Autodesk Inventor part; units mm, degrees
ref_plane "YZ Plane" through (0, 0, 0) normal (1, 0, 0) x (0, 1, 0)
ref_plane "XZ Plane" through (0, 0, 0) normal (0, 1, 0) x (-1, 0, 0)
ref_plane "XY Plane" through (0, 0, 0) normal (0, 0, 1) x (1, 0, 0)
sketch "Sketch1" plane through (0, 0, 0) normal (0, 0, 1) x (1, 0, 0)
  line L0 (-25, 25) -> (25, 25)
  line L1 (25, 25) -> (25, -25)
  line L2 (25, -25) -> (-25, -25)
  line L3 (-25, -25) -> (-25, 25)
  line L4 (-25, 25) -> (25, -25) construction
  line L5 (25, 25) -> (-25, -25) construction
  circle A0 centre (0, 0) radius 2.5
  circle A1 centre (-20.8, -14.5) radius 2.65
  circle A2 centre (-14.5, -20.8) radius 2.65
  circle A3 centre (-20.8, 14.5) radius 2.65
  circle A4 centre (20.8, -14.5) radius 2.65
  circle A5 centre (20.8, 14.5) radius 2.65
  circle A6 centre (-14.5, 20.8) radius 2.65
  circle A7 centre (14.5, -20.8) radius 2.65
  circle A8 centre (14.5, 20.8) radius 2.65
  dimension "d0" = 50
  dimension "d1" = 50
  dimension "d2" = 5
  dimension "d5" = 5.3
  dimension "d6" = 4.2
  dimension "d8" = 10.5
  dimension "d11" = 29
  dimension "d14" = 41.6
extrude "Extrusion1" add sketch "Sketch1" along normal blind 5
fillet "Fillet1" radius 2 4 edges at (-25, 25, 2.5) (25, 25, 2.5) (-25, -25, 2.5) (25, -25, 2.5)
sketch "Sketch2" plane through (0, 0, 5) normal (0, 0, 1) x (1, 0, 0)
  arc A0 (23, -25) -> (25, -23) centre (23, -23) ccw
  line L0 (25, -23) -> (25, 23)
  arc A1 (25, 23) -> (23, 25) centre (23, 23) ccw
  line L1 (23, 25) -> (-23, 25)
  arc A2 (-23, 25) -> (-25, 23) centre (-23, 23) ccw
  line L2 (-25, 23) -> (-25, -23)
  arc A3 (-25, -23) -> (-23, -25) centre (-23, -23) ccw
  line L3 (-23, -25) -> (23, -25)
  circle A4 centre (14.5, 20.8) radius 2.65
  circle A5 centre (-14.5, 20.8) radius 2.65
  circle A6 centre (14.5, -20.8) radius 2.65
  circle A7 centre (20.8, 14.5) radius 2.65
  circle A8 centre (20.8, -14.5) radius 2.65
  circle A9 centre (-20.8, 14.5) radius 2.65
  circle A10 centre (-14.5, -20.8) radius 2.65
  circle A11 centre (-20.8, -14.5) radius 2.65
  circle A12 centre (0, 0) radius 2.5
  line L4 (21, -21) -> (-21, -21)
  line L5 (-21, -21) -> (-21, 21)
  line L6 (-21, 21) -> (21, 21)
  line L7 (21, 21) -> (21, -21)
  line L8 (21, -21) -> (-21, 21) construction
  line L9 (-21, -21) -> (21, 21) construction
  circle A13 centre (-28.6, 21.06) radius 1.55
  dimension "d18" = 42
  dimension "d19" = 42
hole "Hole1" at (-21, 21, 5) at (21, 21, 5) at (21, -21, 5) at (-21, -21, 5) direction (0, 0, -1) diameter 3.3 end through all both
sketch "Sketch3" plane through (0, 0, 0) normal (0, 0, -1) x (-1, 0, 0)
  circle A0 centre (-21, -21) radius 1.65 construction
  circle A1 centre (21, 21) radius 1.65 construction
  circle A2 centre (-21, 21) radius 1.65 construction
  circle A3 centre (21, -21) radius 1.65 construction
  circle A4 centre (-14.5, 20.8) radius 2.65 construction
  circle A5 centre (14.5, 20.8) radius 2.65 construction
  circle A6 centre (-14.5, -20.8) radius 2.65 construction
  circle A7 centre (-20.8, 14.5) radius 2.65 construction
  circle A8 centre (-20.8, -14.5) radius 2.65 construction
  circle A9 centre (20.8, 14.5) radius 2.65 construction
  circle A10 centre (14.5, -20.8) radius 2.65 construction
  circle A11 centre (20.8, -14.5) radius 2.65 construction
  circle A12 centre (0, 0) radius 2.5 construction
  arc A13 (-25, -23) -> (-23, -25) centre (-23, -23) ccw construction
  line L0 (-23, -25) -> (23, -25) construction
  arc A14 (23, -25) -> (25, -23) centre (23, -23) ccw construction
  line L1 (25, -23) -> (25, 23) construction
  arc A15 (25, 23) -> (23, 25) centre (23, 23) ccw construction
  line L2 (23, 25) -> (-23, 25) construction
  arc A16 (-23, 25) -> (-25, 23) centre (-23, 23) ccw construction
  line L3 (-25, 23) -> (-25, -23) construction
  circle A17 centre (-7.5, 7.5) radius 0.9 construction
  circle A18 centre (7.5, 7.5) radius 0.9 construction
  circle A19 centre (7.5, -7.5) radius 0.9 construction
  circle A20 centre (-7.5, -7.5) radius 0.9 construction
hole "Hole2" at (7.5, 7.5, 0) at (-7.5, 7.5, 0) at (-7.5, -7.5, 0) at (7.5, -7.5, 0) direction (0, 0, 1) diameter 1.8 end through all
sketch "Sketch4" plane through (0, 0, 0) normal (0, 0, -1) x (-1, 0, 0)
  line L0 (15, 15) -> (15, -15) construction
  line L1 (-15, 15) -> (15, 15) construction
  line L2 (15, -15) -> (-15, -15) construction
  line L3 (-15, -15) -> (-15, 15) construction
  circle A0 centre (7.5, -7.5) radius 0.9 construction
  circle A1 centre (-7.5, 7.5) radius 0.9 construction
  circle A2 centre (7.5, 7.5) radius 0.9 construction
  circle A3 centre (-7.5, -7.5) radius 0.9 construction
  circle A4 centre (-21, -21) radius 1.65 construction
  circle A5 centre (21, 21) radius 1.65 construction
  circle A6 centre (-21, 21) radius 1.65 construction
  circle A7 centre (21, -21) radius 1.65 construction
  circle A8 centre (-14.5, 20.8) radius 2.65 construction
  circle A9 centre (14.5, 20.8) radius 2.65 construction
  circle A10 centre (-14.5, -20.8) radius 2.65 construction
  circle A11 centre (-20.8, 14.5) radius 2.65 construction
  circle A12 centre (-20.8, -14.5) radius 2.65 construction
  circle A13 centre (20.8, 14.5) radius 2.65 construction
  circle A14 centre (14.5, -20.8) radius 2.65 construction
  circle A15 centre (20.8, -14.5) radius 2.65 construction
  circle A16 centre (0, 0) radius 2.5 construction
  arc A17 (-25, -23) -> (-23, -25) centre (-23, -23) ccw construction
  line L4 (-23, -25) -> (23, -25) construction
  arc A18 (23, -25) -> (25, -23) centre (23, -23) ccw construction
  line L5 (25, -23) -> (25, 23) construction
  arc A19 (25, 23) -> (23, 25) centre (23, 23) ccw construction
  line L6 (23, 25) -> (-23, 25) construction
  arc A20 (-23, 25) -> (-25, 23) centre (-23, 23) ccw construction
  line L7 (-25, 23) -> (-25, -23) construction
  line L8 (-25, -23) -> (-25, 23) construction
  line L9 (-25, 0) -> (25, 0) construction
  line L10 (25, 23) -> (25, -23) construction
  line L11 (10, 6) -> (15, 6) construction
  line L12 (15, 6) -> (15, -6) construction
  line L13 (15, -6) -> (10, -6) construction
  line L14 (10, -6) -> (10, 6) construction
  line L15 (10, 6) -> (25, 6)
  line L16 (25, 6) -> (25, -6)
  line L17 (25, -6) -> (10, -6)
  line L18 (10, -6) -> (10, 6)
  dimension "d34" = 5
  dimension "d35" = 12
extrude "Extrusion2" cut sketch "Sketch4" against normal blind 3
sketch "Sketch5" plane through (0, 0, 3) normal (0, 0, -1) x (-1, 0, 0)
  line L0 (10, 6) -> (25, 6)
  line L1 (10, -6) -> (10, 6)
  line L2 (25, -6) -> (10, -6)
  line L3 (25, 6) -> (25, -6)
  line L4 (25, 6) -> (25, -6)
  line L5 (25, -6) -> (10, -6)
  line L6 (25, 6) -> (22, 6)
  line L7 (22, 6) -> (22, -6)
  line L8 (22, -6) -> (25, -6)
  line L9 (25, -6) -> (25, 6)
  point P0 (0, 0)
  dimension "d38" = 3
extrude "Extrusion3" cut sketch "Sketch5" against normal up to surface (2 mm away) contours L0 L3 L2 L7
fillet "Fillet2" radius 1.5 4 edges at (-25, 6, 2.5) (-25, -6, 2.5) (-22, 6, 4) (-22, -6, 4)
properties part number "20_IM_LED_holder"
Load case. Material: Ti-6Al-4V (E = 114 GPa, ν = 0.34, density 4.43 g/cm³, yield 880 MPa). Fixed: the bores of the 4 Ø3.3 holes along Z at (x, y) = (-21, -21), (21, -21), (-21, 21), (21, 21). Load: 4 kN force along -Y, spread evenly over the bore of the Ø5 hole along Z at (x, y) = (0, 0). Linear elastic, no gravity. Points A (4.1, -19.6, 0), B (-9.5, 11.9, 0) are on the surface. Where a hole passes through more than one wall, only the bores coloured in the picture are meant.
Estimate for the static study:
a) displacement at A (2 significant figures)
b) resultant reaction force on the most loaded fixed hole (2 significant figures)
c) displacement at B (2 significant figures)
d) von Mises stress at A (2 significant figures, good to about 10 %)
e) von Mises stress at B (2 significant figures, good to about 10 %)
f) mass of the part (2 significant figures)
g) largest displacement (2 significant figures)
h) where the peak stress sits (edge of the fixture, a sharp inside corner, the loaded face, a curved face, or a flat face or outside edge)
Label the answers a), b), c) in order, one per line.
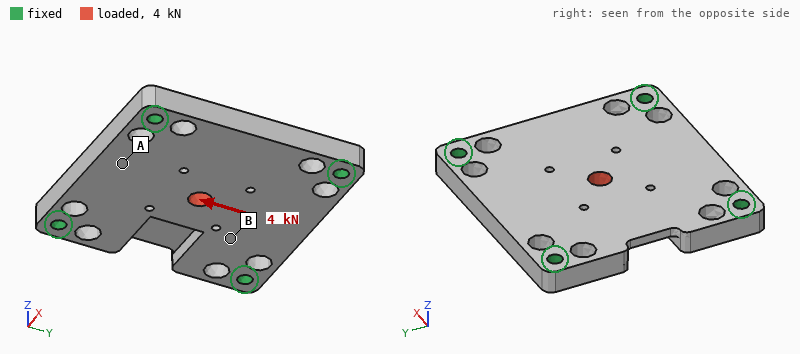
a) 6.2 µm
b) 1.2 kN
c) 5.6 µm
d) 8.9 MPa
e) 20 MPa
f) 47 g
g) 9.4 µm
h) the loaded face
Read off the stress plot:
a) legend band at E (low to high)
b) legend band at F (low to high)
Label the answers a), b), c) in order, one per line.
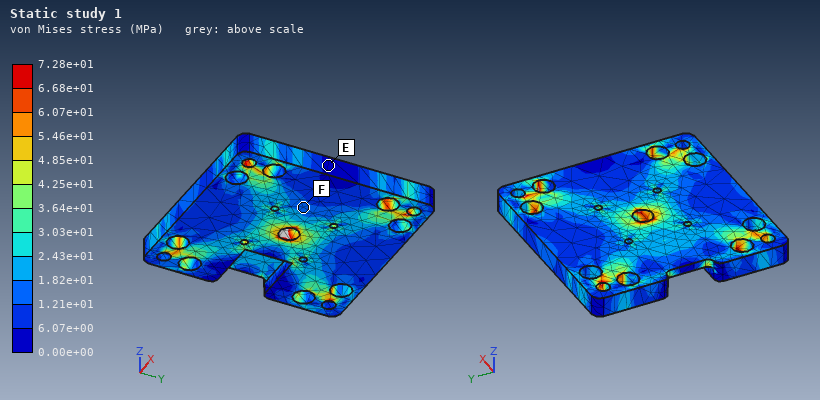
a) 0.00e+00 to 6.07e+00 MPa
b) 1.21e+01 to 1.82e+01 MPa
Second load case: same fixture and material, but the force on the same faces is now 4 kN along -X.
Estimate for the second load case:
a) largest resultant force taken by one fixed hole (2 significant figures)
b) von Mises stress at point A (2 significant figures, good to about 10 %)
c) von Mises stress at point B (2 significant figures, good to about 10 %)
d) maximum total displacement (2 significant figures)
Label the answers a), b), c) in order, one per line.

a) 1.2 kN
b) 7.7 MPa
c) 21 MPa
d) 9.8 µm
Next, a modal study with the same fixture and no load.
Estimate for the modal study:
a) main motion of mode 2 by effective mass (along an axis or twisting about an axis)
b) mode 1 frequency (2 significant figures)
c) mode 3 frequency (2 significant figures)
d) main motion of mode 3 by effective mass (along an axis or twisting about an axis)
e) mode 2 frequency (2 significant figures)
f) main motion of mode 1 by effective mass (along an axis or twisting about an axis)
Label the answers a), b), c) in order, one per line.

a) twisting about X
b) 8000 Hz
c) 14 kHz
d) twisting about Y
e) 13 kHz
f) along Z
